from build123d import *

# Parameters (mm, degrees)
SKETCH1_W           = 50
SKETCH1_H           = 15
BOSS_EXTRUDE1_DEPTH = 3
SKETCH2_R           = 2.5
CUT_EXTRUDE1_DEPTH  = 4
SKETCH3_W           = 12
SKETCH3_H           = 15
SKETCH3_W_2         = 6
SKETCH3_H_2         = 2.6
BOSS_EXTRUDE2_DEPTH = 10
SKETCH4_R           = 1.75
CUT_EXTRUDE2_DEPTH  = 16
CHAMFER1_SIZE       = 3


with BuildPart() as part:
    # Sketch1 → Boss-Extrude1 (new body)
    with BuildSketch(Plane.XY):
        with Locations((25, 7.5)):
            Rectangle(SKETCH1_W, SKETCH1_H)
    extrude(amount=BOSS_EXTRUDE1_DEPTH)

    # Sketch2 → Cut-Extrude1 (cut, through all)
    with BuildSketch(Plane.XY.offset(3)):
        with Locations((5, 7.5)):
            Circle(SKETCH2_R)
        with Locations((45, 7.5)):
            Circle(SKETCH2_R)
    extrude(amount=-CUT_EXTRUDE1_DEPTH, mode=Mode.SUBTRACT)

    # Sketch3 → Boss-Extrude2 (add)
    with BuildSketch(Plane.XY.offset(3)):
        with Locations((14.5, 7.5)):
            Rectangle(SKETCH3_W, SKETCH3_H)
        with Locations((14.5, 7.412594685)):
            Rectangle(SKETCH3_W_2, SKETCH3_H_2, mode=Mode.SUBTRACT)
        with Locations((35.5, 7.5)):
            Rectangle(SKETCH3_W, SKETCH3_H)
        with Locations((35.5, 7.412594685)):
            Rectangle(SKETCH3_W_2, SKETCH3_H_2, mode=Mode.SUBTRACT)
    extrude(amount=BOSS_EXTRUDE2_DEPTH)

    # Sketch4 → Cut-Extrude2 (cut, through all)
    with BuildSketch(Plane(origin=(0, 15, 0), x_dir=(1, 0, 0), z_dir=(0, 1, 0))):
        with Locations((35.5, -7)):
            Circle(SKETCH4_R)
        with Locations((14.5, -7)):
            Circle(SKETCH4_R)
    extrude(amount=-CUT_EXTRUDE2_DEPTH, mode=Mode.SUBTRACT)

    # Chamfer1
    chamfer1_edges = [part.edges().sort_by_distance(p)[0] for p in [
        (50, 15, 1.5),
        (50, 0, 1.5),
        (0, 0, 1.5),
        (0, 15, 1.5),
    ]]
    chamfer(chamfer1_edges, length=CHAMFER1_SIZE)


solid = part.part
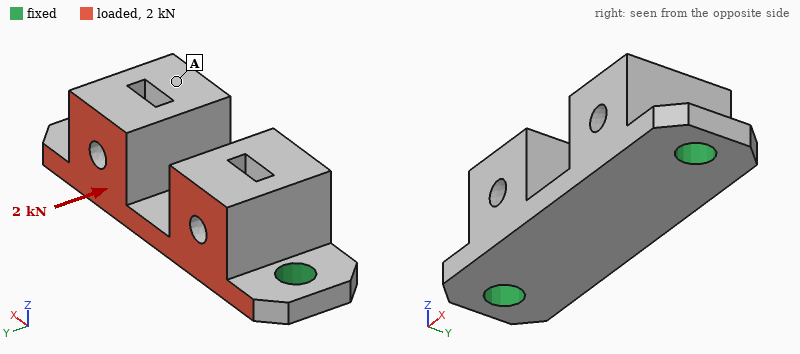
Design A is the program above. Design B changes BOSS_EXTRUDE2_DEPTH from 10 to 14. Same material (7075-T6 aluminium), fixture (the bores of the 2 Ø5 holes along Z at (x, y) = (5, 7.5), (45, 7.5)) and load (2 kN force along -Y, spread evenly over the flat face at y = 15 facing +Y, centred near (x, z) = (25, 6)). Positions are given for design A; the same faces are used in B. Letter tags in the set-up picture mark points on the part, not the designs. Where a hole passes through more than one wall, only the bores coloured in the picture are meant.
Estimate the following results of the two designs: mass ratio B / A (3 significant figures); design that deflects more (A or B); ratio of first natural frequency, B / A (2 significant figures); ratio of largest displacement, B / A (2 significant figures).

1.26
B
0.77
1.7
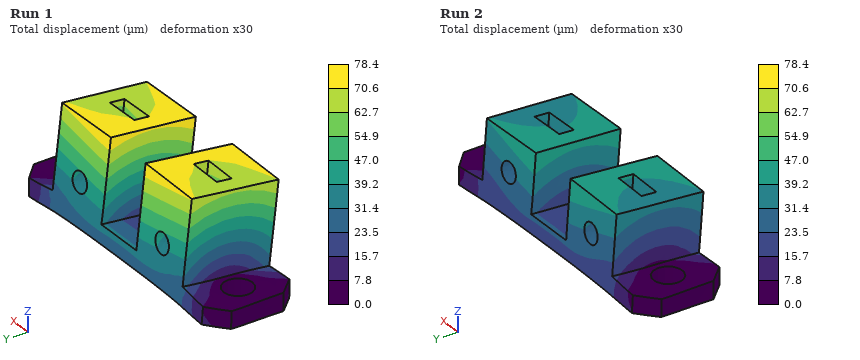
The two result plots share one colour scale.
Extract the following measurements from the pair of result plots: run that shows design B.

Run 1
